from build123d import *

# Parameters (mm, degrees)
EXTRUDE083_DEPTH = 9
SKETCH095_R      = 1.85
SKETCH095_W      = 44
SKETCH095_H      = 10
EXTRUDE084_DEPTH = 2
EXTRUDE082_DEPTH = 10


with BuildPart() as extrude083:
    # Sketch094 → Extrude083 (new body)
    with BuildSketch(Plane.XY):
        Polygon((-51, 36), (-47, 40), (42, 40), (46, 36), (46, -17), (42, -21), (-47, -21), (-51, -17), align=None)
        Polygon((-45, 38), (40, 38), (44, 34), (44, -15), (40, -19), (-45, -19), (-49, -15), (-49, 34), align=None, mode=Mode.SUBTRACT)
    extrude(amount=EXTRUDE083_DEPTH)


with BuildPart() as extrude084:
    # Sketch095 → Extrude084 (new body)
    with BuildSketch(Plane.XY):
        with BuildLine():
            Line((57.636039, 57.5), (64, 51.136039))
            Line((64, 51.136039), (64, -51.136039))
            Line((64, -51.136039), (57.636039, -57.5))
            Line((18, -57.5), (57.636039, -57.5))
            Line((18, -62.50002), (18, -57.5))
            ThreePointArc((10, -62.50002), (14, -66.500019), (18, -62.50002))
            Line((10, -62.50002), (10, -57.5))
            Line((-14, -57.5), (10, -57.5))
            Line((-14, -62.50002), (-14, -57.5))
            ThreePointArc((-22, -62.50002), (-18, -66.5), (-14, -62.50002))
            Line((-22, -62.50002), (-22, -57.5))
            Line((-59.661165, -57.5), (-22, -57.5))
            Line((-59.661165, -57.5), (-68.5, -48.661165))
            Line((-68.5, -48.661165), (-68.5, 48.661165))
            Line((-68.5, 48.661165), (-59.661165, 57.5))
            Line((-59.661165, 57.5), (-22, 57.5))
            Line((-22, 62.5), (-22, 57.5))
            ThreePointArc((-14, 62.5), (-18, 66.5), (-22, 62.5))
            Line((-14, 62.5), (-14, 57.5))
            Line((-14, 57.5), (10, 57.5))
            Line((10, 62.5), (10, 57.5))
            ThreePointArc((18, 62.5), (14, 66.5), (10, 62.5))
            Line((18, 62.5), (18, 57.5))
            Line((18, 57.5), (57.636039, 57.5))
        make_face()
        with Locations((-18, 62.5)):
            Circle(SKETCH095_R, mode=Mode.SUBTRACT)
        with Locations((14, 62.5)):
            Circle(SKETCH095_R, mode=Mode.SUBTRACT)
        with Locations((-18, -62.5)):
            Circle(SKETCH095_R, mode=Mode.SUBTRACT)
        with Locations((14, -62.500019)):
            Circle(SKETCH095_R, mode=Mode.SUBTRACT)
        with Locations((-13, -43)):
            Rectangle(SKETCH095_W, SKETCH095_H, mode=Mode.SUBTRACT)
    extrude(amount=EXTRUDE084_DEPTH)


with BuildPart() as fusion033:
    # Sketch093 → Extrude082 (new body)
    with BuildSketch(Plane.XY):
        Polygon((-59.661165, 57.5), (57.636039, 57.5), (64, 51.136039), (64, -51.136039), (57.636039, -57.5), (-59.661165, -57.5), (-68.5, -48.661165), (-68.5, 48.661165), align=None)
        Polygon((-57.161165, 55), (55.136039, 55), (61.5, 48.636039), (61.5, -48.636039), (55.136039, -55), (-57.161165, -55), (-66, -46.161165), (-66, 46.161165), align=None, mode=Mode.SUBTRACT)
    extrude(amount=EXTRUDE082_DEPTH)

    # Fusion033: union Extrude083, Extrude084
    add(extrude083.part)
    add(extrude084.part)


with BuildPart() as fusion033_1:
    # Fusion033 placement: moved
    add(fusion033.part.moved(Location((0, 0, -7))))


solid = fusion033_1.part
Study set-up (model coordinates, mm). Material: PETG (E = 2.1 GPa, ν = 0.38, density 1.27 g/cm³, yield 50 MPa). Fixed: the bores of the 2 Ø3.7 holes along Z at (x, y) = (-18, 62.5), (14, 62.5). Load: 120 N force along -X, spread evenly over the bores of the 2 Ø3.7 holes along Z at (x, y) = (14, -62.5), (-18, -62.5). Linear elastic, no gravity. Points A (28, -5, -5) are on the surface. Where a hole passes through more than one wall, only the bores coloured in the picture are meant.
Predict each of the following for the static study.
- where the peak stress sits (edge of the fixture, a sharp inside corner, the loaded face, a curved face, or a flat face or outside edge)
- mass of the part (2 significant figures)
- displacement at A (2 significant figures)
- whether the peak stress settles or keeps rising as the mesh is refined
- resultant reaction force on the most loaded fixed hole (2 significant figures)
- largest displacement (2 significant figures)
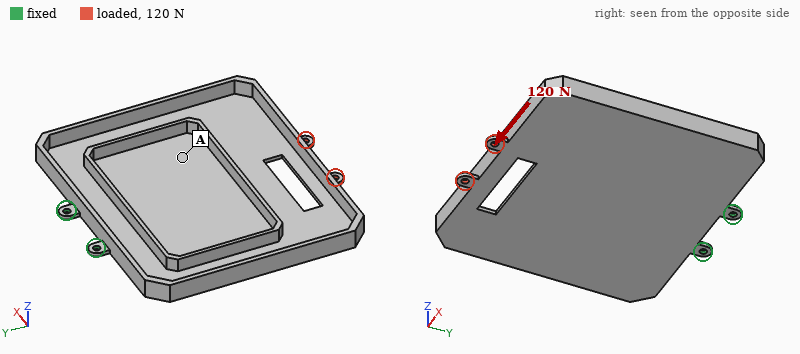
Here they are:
edge of the fixture
56 g
1.0 mm
keeps rising
450 N
2.0 mm
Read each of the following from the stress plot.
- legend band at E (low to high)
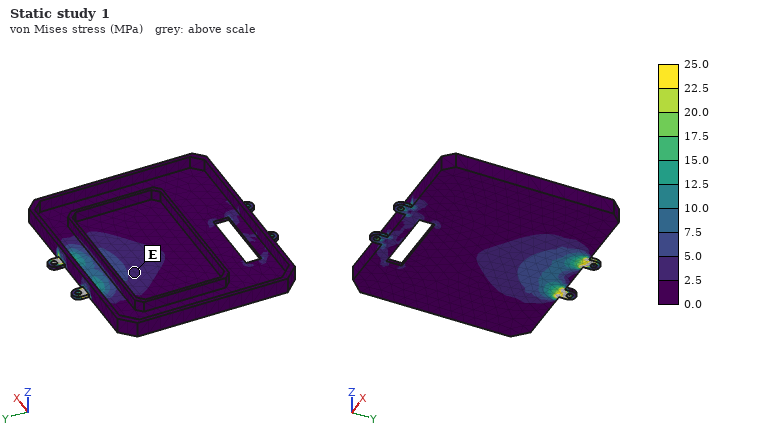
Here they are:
2.5 to 5.0 MPa
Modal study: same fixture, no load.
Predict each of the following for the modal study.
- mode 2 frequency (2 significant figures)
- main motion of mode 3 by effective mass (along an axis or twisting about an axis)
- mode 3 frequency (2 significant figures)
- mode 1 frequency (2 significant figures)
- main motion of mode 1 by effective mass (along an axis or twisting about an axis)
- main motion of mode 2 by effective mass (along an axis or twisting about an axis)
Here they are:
55 Hz
along Z
260 Hz
19 Hz
along Z
twisting about Y
